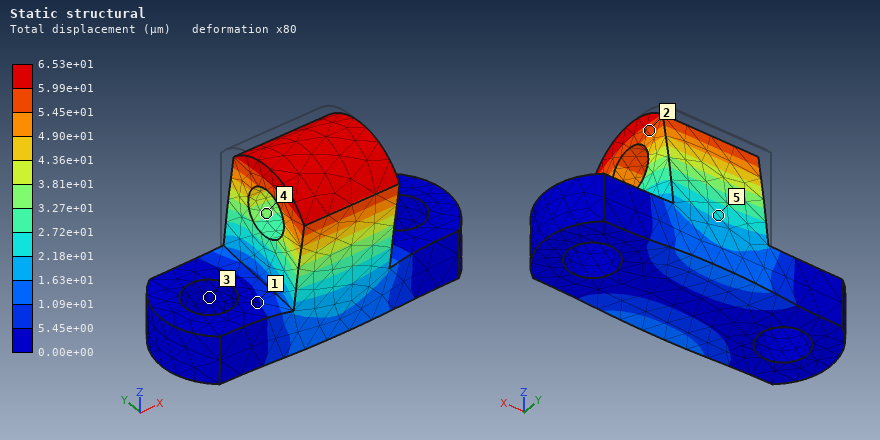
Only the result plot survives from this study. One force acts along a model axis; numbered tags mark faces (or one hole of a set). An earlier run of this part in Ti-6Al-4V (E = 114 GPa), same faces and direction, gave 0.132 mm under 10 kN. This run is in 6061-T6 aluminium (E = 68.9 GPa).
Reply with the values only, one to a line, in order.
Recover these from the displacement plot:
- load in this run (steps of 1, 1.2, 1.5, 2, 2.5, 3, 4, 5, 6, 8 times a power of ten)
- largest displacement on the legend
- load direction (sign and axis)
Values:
3 kN
6.53e+01 µm
-Y
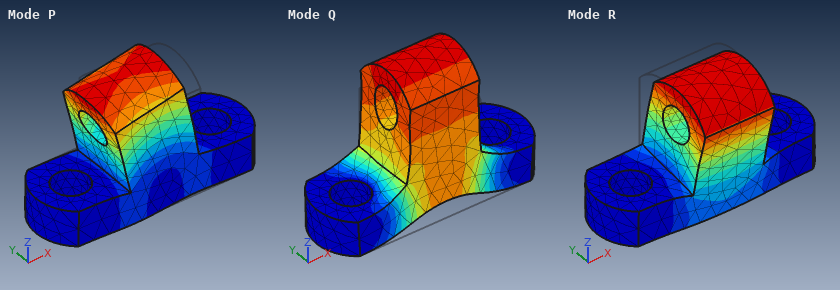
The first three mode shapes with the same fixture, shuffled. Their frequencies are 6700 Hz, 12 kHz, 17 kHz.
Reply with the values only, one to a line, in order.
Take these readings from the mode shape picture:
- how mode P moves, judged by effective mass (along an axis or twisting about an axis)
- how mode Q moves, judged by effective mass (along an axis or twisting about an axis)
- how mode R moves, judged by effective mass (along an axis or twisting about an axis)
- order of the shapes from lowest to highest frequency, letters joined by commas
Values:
along X
along Z
along Y
R, P, Q
